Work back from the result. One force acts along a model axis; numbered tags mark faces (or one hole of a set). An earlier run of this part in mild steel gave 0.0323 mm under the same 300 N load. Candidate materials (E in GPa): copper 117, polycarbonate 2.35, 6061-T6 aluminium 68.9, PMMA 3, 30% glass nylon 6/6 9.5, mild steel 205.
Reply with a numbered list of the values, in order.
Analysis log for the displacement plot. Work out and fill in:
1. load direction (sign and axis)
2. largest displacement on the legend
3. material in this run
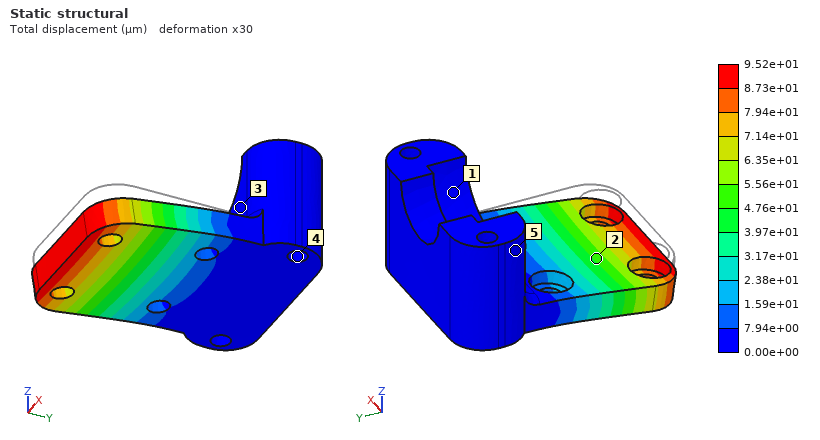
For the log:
1. -Z
2. 9.52e+01 µm
3. 6061-T6 aluminium
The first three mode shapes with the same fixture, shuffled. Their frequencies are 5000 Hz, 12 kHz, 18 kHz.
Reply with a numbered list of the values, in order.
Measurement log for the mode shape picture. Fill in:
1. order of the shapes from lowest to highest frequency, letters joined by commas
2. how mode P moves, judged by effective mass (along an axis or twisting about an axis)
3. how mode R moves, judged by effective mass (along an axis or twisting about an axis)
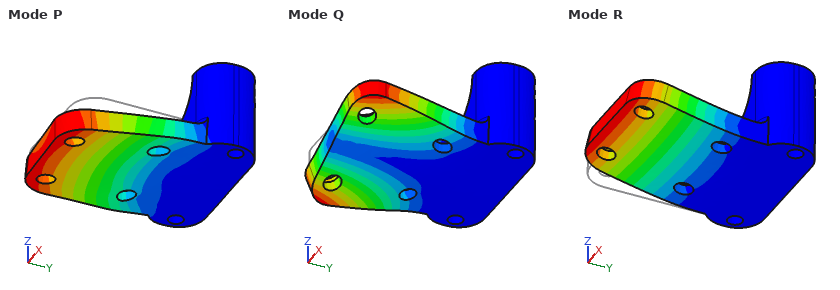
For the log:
1. R, Q, P
2. along X
3. along Z
